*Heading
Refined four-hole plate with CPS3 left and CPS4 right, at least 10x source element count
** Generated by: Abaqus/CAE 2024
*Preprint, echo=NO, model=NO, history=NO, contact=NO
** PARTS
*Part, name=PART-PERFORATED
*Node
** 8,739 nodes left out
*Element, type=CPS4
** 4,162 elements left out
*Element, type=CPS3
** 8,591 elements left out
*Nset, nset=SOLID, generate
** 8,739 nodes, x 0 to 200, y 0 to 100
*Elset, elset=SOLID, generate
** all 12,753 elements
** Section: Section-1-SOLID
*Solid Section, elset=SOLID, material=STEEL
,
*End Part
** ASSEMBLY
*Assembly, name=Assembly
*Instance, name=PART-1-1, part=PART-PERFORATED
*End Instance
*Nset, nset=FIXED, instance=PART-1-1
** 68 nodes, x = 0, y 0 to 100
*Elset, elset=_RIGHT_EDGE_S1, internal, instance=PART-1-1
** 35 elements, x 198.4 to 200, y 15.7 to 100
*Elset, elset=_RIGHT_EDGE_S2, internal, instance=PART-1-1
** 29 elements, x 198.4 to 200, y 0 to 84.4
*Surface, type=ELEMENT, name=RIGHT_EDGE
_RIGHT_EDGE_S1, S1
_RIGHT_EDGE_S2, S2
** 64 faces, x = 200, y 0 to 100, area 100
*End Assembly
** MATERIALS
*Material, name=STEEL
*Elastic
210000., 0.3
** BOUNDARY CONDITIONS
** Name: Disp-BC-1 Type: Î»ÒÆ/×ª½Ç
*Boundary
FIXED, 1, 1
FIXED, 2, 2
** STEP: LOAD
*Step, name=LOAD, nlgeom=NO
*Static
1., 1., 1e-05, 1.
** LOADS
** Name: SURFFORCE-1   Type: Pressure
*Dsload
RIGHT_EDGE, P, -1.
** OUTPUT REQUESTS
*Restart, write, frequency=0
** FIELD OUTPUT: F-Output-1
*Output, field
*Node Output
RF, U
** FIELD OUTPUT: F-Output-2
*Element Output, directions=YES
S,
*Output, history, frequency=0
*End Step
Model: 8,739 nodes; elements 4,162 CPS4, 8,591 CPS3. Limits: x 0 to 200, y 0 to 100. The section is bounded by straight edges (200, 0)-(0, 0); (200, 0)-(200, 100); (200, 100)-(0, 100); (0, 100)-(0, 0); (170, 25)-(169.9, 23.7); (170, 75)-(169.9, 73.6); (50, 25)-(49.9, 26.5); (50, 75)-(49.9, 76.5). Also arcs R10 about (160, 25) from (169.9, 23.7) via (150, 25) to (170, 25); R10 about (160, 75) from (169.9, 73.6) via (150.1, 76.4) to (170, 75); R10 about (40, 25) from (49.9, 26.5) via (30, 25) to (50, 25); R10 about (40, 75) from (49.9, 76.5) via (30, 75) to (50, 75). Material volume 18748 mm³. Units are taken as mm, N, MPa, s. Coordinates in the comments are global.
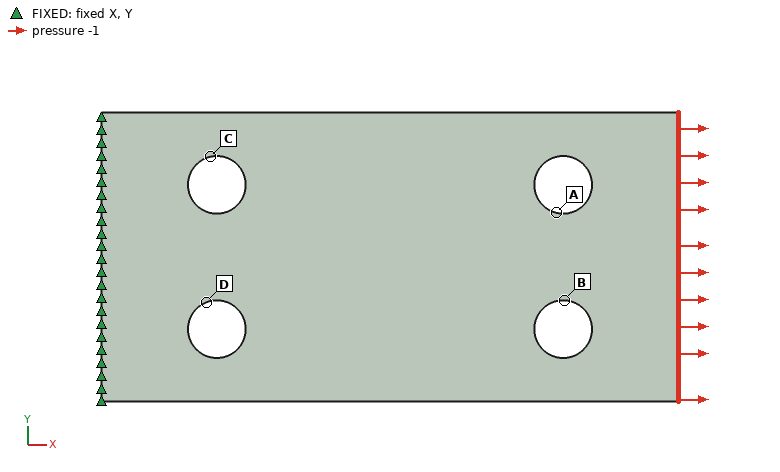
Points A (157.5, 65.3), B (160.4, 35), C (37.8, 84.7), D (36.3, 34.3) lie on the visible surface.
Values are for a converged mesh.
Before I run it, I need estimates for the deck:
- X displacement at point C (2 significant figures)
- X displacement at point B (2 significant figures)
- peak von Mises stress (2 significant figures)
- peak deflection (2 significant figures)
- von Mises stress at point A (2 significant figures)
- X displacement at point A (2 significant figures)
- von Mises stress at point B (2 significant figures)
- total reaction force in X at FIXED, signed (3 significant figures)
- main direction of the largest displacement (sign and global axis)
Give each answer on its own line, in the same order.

2.0e-04 mm
9.2e-04 mm
3.6 MPa
0.0012 mm
3.1 MPa
8.7e-04 mm
3.3 MPa
-100 N
+X
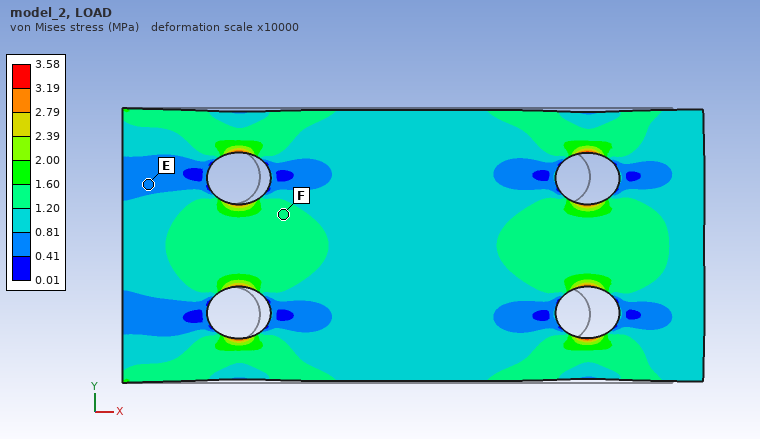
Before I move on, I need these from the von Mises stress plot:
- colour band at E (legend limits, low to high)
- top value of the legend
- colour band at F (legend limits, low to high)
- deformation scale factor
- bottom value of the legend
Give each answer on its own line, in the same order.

0.41 to 0.81 MPa
3.58 MPa
1.20 to 1.60 MPa
10000
0.01 MPa
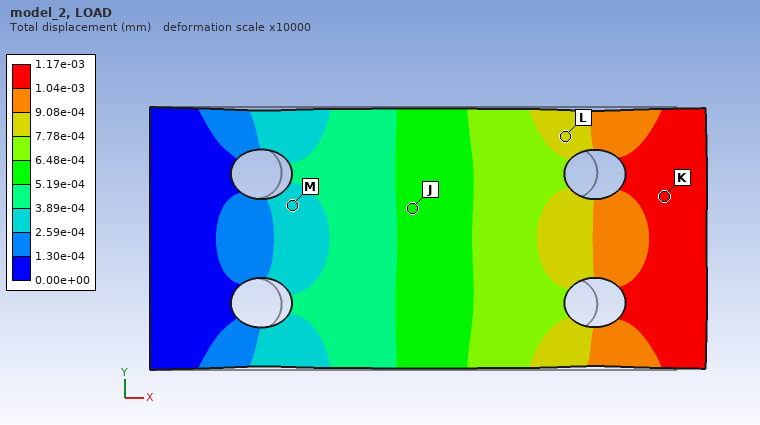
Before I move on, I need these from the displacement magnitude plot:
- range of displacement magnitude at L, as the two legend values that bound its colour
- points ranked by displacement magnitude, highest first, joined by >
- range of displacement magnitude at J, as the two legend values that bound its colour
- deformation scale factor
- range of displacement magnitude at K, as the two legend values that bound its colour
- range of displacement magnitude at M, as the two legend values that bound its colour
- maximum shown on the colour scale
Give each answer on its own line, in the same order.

7.78e-04 to 9.08e-04 mm
K > L > J > M
5.19e-04 to 6.48e-04 mm
10000
1.04e-03 to 1.17e-03 mm
2.59e-04 to 3.89e-04 mm
1.17e-03 mm
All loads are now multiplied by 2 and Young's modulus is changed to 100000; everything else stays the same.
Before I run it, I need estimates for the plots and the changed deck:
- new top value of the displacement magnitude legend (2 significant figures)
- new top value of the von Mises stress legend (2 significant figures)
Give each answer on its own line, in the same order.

0.0049 mm
7.2 MPa
